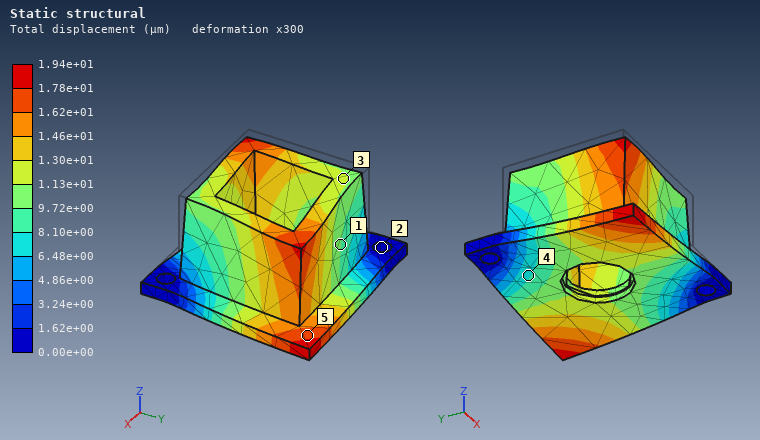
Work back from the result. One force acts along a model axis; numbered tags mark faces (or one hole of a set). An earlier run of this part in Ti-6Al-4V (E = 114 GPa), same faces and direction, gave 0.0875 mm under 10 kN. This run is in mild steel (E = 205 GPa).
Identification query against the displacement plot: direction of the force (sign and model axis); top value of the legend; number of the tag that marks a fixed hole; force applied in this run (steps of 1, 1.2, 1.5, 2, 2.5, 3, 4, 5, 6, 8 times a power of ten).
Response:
-Z
1.94e+01 µm
2
4 kN
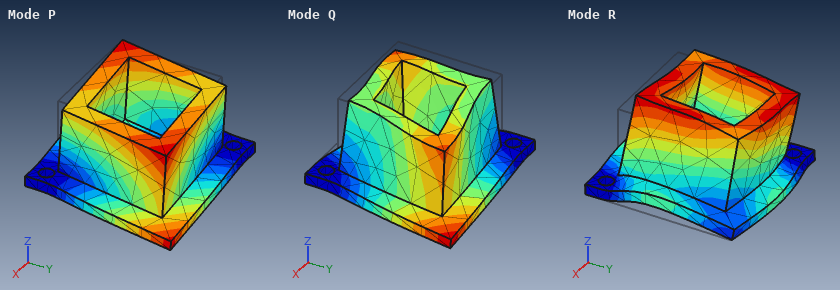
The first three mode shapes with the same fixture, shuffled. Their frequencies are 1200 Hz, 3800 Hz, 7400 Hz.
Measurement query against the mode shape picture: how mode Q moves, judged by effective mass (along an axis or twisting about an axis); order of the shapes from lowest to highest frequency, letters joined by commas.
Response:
along Z
P, Q, R
